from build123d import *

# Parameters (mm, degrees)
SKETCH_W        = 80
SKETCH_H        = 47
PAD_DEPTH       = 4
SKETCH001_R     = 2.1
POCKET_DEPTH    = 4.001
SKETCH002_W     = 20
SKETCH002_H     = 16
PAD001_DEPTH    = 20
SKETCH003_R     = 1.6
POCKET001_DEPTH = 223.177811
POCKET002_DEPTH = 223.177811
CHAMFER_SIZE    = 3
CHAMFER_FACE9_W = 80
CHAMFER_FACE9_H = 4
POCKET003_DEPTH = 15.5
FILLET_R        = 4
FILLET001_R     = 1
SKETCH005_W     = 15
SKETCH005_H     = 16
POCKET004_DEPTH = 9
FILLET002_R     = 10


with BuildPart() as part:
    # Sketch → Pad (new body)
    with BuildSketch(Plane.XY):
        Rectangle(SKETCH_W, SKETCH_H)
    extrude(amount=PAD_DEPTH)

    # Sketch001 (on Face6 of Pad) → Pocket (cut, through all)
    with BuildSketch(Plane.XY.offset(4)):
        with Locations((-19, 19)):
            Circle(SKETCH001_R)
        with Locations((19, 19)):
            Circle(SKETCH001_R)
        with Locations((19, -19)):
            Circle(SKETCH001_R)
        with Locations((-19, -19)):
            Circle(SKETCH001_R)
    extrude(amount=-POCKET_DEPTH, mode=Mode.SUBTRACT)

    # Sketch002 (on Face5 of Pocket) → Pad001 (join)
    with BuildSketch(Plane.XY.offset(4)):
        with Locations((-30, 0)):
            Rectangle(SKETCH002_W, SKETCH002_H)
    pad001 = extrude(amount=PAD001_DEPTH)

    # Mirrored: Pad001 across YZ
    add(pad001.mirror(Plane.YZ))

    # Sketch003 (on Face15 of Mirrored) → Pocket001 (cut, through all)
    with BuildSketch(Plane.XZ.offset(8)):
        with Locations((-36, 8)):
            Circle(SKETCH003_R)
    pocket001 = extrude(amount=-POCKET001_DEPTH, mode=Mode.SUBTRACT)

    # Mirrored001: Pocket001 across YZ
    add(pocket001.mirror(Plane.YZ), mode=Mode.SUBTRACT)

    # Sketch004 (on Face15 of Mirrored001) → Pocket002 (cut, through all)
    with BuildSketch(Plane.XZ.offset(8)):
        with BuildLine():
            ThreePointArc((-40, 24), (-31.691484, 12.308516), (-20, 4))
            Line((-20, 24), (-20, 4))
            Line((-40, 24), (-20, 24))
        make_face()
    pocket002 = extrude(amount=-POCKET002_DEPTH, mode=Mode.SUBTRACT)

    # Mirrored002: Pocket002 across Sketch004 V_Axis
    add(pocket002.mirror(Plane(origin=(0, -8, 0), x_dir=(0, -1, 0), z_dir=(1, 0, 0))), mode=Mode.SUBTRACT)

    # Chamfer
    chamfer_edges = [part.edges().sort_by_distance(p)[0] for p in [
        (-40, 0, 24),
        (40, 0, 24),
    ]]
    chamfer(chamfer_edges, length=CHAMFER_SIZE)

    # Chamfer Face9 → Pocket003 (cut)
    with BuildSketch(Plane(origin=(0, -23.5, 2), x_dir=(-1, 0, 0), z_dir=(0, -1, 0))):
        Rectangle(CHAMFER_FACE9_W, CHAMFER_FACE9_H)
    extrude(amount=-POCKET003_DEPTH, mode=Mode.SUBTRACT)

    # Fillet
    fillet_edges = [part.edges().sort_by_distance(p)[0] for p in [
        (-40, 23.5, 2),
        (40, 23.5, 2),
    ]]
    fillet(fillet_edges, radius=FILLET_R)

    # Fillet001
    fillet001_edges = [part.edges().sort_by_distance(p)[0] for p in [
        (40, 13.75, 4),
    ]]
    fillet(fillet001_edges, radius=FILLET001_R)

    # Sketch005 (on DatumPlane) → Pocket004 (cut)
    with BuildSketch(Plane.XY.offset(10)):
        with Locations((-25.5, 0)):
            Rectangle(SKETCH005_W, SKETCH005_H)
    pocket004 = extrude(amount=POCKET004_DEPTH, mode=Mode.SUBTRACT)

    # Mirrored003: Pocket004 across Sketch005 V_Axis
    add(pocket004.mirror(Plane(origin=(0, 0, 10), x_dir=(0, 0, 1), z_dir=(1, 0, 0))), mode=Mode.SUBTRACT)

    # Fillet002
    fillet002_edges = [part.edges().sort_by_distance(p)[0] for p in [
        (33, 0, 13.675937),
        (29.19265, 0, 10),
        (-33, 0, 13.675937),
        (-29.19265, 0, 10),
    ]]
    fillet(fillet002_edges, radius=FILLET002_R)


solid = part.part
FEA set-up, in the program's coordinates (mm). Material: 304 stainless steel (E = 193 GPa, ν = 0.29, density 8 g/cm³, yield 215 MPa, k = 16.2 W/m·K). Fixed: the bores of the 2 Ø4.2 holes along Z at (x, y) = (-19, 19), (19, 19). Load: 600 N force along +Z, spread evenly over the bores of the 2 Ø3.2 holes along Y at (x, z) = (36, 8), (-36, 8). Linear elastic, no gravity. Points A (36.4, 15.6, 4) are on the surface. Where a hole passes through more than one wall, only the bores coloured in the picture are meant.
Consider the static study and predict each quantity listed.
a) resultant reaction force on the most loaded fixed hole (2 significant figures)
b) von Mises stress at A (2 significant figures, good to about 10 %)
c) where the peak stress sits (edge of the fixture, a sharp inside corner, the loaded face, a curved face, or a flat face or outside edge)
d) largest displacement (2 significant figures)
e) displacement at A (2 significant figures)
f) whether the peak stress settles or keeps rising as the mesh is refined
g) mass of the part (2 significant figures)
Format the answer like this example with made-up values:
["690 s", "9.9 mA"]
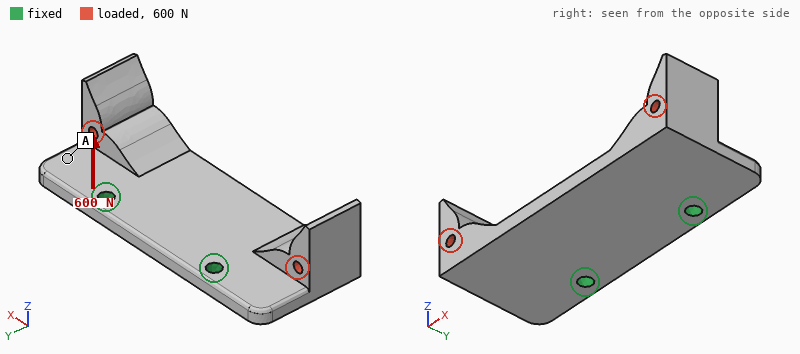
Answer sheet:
["300 N", "22 MPa", "edge of the fixture", "90 µm", "21 µm", "keeps rising", "110 g"]
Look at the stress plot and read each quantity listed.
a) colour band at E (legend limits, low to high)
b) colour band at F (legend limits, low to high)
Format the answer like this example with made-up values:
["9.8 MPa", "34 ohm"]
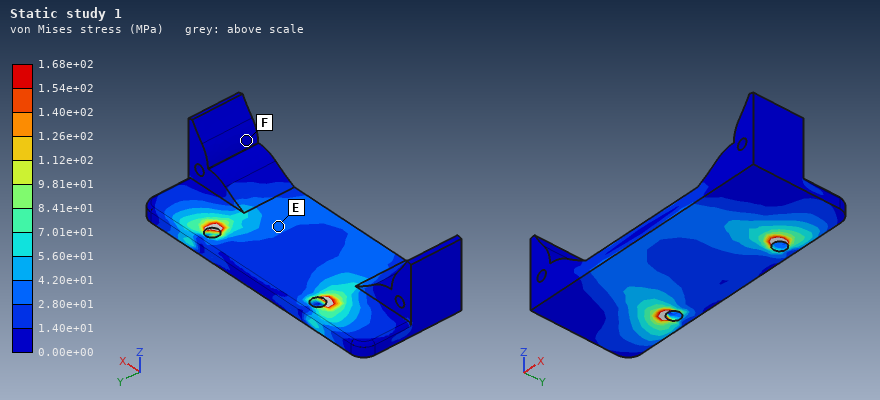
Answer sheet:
["2.80e+01 to 4.20e+01 MPa", "0.00e+00 to 1.40e+01 MPa"]
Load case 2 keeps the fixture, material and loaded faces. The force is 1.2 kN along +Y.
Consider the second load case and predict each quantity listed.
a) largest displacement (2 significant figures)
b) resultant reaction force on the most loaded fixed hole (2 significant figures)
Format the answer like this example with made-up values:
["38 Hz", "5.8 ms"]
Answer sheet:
["54 µm", "730 N"]
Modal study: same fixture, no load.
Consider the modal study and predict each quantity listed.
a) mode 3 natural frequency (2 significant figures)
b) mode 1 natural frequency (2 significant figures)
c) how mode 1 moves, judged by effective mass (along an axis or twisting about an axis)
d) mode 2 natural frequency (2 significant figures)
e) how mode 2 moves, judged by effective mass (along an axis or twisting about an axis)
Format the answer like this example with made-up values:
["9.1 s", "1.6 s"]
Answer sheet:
["4000 Hz", "2200 Hz", "along Z", "2300 Hz", "twisting about Y"]
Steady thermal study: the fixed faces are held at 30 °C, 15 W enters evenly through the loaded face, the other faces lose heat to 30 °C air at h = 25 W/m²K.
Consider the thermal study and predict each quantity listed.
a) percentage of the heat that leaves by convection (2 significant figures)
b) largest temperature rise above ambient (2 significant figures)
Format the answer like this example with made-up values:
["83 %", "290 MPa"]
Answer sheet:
["46 %", "76 K"]
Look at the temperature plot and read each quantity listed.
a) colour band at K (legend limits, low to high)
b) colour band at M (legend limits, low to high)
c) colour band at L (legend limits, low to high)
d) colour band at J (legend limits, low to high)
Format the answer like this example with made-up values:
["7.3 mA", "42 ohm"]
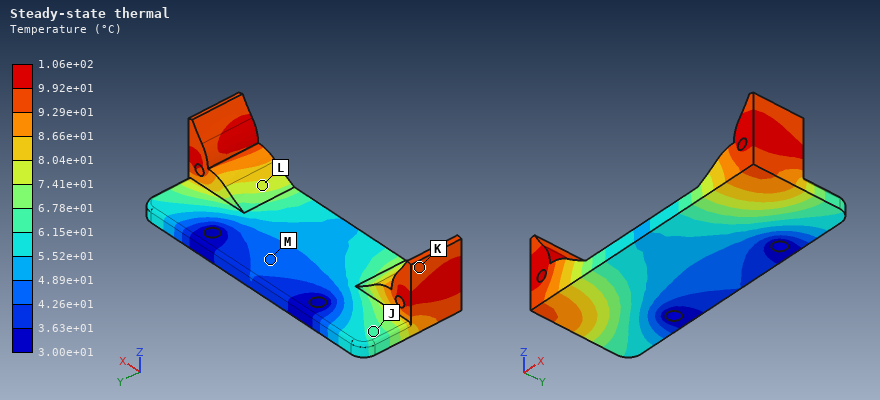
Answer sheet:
["9.29e+01 to 9.92e+01 °C", "4.26e+01 to 4.89e+01 °C", "7.41e+01 to 8.04e+01 °C", "6.15e+01 to 6.78e+01 °C"]
